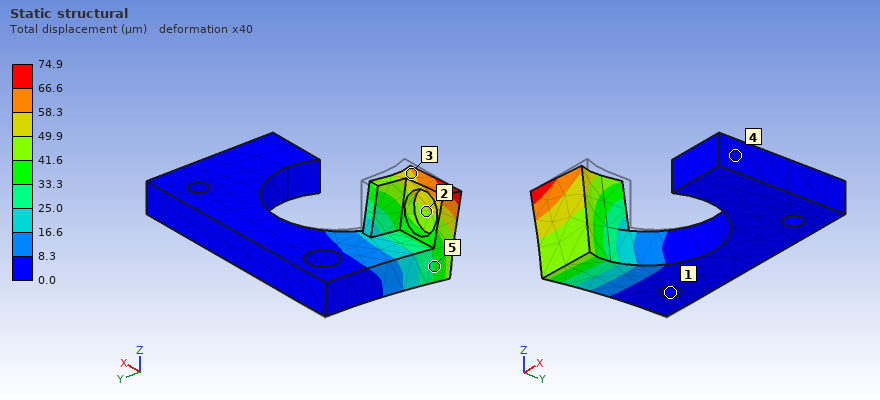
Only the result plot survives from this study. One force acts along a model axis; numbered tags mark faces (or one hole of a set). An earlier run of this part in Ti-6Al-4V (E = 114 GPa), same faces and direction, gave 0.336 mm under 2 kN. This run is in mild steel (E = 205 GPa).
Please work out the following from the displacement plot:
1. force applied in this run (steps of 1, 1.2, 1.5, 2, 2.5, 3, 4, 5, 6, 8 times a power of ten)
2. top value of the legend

800 N
74.9 µm
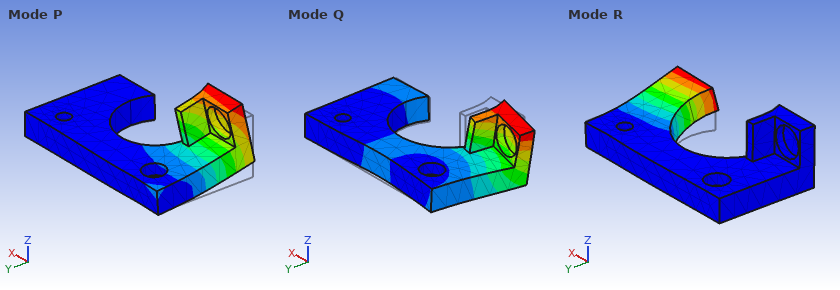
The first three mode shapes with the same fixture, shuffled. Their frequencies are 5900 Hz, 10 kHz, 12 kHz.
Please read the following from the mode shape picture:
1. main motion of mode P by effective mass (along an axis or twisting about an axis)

along Z
